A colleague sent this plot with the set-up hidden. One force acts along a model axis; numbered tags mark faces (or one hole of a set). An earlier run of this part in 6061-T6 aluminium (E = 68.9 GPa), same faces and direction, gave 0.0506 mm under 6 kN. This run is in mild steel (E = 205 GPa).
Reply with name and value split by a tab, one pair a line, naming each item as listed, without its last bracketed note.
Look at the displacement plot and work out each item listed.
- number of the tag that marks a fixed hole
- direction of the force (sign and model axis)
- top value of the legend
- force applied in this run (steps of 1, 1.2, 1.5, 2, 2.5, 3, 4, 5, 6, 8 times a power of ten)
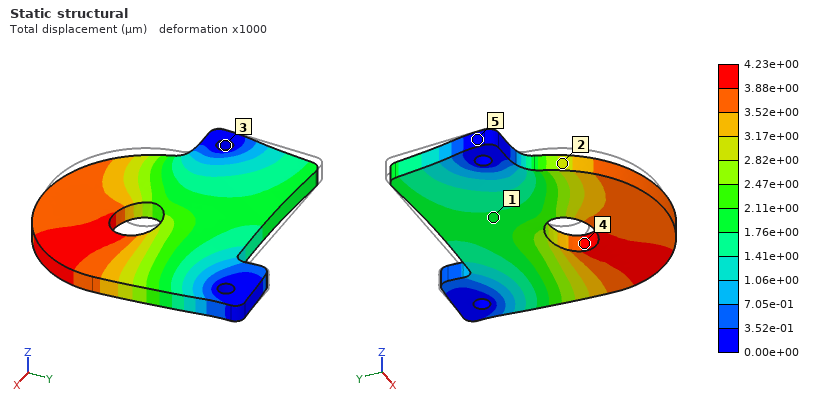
number of the tag that marks a fixed hole	3
direction of the force	+X
top value of the legend	4.23e+00 µm
force applied in this run	1.5 kN
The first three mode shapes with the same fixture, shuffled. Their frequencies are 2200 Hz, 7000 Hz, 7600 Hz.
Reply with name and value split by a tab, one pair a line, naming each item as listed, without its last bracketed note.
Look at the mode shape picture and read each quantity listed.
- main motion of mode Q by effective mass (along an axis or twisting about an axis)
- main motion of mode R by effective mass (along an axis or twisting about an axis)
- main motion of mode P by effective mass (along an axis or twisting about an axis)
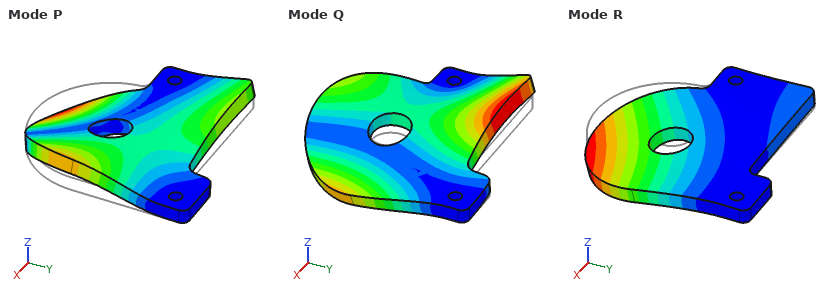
main motion of mode Q by effective mass	along Z
main motion of mode R by effective mass	along Z
main motion of mode P by effective mass	along Z
